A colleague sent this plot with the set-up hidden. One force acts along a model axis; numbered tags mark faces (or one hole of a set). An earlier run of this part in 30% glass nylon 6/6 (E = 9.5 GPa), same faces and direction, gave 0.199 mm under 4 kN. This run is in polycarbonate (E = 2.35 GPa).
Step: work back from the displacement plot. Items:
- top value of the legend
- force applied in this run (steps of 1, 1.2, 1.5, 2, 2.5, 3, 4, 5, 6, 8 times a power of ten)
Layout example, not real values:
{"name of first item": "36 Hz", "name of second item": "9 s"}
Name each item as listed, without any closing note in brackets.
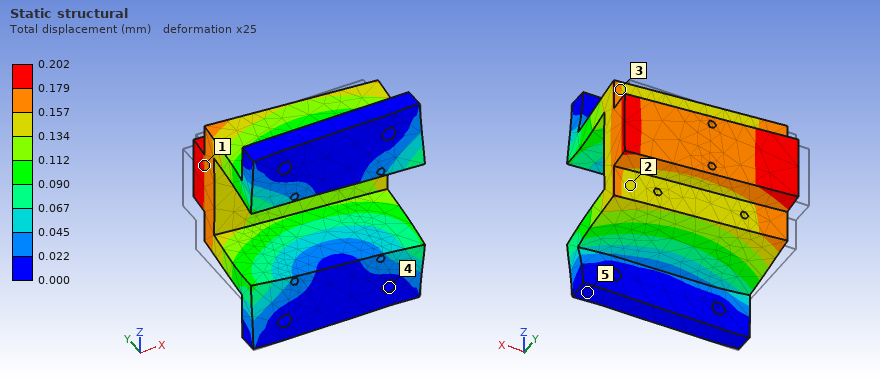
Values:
{"top value of the legend": "0.202 mm", "force applied in this run": "1 kN"}
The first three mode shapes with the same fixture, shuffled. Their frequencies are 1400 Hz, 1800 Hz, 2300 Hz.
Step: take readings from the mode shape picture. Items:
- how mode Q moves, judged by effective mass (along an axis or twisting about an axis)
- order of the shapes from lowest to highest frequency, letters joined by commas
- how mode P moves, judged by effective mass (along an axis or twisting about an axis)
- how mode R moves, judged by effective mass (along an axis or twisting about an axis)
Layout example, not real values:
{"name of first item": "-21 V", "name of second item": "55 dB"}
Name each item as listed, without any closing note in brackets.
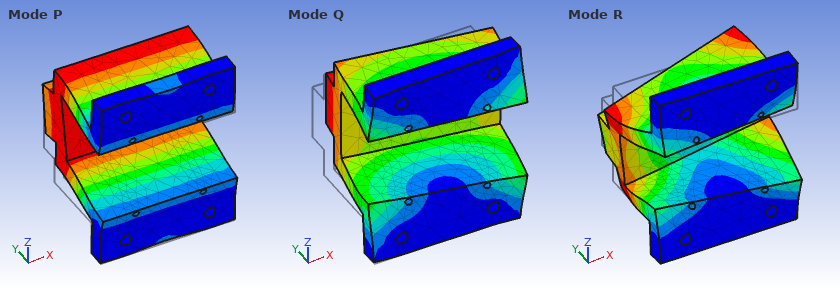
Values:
{"how mode Q moves, judged by effective mass": "along X", "order of the shapes from lowest to highest frequency, letters joined by commas": "P, Q, R", "how mode P moves, judged by effective mass": "along Z", "how mode R moves, judged by effective mass": "twisting about Y"}
